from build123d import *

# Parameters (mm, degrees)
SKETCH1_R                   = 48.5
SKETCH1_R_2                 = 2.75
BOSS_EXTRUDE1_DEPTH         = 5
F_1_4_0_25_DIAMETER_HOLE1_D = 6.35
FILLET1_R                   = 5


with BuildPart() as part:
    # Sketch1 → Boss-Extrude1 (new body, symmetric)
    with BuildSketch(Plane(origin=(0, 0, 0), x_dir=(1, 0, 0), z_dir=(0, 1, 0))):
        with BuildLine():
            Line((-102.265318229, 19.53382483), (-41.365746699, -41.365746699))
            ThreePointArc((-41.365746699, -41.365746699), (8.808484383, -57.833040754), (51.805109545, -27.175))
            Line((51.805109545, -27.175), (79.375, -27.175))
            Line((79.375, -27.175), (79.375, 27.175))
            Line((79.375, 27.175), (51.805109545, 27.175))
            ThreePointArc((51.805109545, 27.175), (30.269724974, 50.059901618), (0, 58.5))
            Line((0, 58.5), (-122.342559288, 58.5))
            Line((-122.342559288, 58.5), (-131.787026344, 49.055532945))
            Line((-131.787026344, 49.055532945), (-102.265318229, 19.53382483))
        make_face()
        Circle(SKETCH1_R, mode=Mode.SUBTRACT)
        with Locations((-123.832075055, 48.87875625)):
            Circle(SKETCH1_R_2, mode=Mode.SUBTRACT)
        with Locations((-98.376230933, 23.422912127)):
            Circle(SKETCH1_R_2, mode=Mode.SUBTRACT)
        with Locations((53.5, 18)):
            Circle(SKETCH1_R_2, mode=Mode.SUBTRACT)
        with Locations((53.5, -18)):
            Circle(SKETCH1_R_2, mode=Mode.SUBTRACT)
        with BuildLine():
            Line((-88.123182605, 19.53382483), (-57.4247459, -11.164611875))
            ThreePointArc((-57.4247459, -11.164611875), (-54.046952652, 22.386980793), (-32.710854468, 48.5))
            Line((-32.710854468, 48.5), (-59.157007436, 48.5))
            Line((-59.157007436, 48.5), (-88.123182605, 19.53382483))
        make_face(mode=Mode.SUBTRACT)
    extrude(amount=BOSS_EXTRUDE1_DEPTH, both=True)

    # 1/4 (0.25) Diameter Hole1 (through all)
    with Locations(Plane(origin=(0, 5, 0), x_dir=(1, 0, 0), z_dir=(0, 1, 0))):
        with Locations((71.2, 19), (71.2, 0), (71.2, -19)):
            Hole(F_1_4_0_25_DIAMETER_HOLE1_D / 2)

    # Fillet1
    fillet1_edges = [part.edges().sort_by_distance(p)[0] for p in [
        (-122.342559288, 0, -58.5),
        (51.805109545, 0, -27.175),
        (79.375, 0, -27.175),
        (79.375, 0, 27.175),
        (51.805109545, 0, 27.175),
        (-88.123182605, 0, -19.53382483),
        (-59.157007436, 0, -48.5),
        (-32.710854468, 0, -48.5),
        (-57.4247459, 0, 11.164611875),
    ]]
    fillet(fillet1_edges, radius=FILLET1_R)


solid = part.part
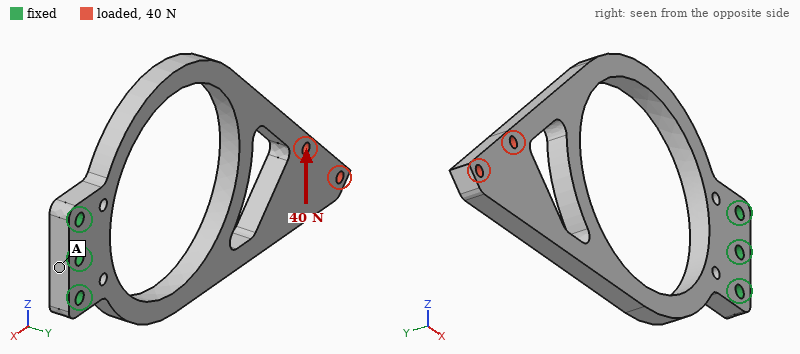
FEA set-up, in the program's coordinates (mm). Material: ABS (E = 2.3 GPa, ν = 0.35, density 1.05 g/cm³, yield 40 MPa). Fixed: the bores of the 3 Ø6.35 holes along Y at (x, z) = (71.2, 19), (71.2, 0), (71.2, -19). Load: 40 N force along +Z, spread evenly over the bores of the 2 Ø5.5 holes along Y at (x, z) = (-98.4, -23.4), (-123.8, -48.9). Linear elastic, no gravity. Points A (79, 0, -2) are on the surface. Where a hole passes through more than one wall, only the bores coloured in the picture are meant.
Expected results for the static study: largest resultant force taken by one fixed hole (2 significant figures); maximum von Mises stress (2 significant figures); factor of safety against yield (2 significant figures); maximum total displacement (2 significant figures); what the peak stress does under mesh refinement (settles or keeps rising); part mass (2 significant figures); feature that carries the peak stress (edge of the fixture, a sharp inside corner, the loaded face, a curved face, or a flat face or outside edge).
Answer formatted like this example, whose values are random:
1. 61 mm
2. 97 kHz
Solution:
1. 180 N
2. 14 MPa
3. 2.9
4. 2.7 mm
5. settles
6. 77 g
7. a curved face
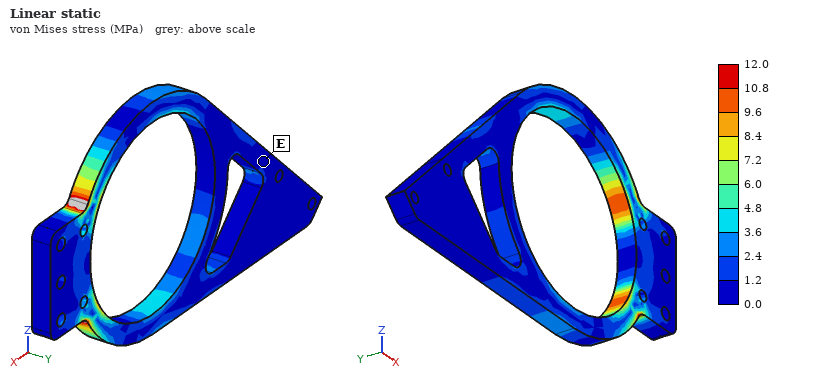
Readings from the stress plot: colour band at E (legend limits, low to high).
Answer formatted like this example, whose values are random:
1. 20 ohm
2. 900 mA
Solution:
1. 0.0 to 1.2 MPa
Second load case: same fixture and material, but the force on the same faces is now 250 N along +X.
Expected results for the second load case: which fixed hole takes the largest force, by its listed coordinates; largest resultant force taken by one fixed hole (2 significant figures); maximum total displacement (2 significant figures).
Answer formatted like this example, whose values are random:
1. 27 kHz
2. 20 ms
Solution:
1. (71.2, -19)
2. 390 N
3. 2.7 mm
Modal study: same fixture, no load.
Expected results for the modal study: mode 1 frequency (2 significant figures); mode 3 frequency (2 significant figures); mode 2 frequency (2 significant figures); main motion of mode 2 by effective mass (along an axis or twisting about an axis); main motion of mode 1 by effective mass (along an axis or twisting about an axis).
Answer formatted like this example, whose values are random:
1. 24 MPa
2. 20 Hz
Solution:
1. 43 Hz
2. 190 Hz
3. 110 Hz
4. along Z
5. along Y
